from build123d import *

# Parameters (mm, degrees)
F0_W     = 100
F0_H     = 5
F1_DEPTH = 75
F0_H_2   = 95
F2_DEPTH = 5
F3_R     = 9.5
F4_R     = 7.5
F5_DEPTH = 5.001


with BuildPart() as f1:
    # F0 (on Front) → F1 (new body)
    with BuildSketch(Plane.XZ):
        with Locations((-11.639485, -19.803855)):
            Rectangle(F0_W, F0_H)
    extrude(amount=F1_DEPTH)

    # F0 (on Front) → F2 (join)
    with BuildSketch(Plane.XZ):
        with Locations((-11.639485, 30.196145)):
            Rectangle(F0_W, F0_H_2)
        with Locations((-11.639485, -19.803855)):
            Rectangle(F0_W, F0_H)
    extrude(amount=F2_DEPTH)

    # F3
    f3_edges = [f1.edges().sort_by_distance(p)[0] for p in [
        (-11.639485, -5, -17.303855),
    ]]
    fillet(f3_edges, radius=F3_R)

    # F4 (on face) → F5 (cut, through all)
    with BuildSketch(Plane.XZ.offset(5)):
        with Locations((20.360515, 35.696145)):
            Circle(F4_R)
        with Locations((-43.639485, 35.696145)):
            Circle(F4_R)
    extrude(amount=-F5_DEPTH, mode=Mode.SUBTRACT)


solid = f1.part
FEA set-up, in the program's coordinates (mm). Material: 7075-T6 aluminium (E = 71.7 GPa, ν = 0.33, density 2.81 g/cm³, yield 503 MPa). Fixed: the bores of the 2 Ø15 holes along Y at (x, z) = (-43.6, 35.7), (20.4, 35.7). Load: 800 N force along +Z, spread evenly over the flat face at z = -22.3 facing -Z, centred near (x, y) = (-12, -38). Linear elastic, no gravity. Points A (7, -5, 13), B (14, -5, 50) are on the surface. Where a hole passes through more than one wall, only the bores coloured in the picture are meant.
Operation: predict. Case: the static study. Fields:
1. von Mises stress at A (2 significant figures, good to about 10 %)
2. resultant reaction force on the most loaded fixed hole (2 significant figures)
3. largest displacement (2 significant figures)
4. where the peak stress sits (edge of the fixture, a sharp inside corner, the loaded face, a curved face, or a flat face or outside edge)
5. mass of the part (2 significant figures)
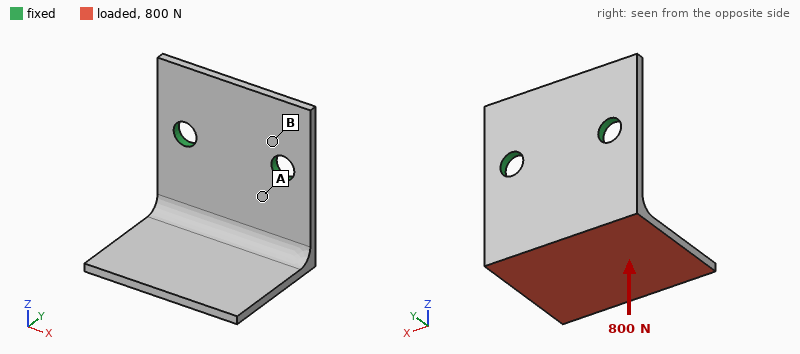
61 MPa
410 N
1.5 mm
a flat face or outside edge
240 g
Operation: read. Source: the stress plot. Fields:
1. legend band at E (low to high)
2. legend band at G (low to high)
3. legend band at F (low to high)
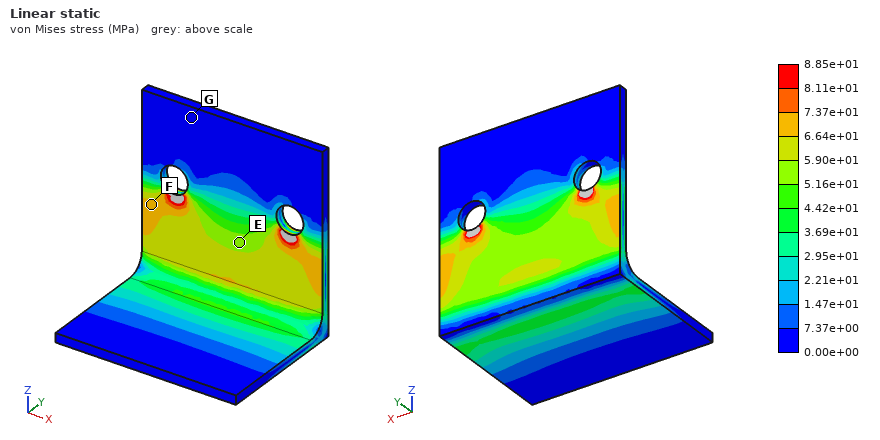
5.16e+01 to 5.90e+01 MPa
0.00e+00 to 7.37e+00 MPa
6.64e+01 to 7.37e+01 MPa
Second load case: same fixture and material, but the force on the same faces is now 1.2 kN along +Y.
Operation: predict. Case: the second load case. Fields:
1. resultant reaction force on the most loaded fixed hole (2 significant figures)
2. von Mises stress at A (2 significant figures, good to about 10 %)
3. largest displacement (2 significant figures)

600 N
90 MPa
1.8 mm
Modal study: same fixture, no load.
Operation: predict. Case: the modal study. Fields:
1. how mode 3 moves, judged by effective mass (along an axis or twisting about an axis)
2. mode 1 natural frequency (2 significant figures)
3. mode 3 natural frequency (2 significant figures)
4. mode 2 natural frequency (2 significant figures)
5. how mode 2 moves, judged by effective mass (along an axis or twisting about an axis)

along Y
380 Hz
1100 Hz
760 Hz
along X
